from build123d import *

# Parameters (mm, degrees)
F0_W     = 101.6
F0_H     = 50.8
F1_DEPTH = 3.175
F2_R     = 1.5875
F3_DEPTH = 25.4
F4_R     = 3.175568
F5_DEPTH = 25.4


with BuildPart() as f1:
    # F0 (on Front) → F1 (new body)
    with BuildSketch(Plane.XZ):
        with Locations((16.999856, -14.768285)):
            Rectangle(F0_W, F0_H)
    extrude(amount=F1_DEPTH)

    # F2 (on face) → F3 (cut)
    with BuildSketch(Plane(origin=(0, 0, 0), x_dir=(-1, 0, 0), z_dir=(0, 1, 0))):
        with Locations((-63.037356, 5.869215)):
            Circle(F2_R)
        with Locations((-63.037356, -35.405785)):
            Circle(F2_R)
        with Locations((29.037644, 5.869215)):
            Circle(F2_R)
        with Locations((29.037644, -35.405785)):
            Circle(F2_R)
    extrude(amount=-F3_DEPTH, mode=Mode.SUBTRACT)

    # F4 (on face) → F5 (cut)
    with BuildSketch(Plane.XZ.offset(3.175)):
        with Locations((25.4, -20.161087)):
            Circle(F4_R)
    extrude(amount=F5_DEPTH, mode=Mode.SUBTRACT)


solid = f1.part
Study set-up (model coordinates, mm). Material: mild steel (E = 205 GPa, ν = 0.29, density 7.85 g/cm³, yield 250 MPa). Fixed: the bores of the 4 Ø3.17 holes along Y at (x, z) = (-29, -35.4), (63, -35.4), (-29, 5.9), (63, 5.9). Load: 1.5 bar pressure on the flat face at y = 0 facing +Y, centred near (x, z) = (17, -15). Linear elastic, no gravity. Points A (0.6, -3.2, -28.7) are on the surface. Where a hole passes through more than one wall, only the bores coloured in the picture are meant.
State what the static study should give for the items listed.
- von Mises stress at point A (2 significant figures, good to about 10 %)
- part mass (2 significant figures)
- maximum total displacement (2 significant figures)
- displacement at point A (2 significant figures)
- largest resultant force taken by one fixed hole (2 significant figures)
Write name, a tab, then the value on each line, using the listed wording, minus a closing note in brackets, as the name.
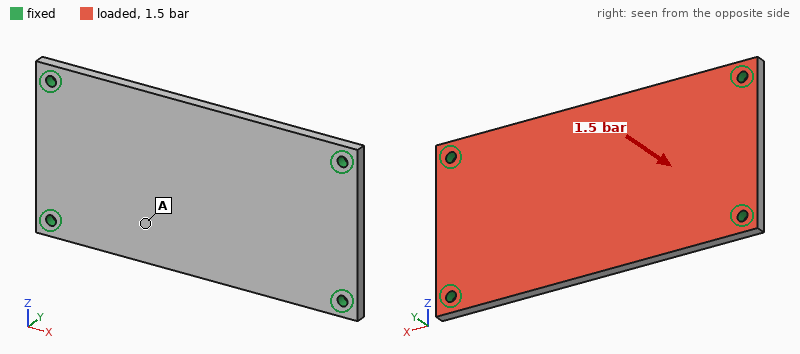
von Mises stress at point A	24 MPa
part mass	130 g
maximum total displacement	68 µm
displacement at point A	52 µm
largest resultant force taken by one fixed hole	190 N
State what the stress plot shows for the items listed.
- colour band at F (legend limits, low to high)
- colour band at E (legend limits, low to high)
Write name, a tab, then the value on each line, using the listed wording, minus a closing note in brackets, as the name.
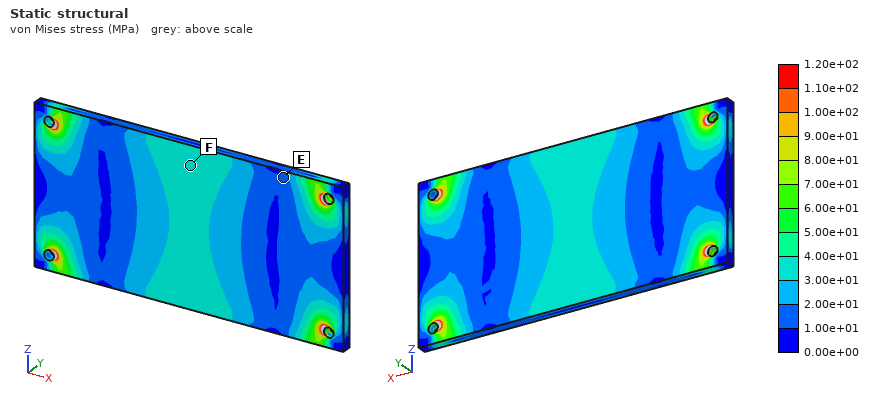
colour band at F	3.00e+01 to 4.00e+01 MPa
colour band at E	1.00e+01 to 2.00e+01 MPa
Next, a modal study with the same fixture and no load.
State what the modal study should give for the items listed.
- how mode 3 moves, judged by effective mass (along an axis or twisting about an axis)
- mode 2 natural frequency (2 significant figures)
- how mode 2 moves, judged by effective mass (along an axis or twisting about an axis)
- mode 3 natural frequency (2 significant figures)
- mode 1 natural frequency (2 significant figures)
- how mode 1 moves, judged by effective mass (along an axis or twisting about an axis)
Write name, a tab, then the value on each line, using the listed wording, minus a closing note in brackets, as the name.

how mode 3 moves, judged by effective mass	twisting about Z
mode 2 natural frequency	3000 Hz
how mode 2 moves, judged by effective mass	twisting about X
mode 3 natural frequency	4700 Hz
mode 1 natural frequency	1700 Hz
how mode 1 moves, judged by effective mass	along Y
